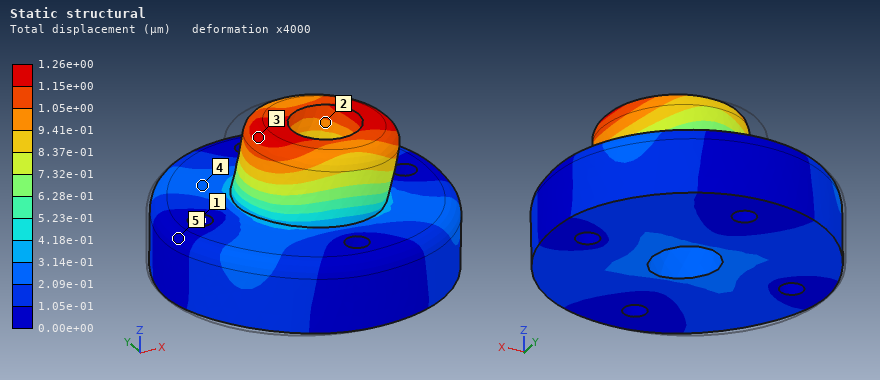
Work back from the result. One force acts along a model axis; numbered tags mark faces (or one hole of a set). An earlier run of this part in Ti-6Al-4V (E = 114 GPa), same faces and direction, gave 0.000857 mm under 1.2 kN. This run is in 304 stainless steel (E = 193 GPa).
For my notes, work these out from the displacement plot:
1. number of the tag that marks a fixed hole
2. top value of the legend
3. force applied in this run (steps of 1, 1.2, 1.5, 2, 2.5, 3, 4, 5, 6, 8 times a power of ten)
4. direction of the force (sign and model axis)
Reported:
1
1.26e+00 µm
3 kN
+X
